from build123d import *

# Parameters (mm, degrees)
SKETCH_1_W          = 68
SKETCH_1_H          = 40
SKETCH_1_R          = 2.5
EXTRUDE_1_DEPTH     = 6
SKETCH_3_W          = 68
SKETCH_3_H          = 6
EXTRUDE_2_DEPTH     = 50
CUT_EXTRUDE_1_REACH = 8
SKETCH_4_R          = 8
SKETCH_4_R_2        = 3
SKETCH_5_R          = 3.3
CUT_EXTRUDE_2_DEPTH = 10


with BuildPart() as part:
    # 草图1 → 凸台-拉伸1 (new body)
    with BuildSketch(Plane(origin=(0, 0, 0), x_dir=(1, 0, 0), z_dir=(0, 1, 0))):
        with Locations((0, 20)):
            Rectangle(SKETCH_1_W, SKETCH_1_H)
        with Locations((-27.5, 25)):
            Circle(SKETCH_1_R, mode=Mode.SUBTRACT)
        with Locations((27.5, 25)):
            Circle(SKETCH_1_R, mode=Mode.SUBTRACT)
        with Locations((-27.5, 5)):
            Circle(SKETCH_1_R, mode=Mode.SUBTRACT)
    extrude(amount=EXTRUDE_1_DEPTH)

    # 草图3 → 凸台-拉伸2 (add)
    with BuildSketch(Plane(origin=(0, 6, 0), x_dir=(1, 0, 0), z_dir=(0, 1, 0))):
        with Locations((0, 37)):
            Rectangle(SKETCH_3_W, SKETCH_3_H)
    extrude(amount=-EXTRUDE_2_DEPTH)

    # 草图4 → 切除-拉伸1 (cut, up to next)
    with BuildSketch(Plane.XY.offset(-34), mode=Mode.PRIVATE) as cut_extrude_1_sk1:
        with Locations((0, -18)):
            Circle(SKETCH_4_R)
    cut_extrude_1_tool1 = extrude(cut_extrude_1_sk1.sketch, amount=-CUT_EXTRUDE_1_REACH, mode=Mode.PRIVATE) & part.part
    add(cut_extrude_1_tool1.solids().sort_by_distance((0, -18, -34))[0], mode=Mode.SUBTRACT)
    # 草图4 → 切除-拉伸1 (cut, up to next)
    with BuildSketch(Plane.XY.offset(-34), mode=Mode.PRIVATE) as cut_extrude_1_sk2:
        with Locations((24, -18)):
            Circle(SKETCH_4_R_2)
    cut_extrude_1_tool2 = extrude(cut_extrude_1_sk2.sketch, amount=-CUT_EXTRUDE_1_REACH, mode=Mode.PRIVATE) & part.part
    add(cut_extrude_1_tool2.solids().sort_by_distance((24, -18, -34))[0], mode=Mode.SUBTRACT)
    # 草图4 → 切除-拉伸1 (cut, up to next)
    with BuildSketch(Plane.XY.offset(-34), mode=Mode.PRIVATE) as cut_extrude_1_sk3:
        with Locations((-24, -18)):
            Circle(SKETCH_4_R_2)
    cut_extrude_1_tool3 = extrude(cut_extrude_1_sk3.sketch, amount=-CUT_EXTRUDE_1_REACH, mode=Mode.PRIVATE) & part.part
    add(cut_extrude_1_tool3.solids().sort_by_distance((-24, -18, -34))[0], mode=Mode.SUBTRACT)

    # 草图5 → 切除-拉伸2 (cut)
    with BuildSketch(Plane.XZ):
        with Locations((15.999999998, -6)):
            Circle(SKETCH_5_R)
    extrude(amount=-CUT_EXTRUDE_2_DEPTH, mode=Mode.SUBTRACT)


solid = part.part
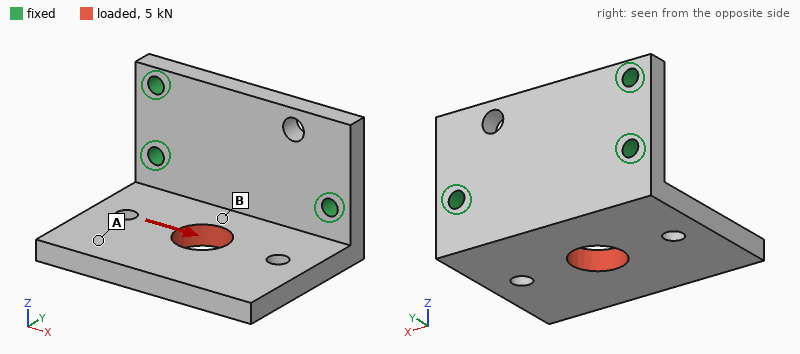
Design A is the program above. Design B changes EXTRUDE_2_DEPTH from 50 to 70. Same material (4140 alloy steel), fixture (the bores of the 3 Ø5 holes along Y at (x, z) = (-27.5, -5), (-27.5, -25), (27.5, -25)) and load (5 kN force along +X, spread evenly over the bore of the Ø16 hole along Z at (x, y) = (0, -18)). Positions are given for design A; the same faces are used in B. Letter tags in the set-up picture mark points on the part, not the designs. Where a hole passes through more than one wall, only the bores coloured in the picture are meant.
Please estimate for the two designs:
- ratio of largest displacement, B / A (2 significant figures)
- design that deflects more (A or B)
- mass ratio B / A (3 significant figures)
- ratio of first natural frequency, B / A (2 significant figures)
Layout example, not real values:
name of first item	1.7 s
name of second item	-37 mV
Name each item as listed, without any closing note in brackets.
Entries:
ratio of largest displacement, B / A	1.2
design that deflects more	B
mass ratio B / A	1.25
ratio of first natural frequency, B / A	0.52
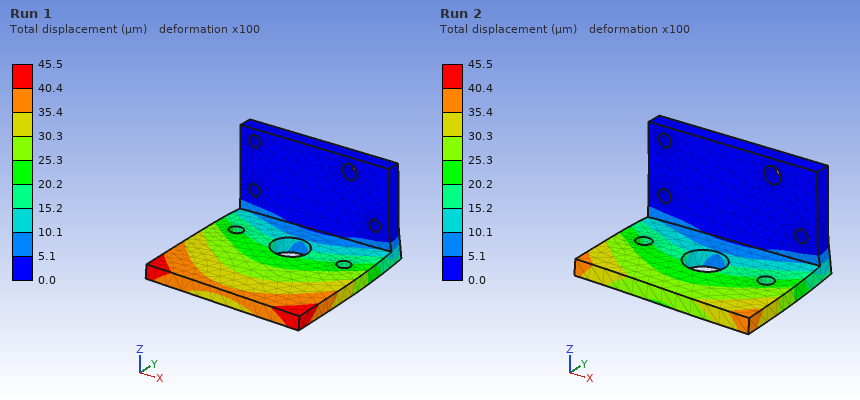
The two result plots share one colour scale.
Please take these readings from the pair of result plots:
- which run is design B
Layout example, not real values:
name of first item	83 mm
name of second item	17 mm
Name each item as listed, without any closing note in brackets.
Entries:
which run is design B	Run 1
